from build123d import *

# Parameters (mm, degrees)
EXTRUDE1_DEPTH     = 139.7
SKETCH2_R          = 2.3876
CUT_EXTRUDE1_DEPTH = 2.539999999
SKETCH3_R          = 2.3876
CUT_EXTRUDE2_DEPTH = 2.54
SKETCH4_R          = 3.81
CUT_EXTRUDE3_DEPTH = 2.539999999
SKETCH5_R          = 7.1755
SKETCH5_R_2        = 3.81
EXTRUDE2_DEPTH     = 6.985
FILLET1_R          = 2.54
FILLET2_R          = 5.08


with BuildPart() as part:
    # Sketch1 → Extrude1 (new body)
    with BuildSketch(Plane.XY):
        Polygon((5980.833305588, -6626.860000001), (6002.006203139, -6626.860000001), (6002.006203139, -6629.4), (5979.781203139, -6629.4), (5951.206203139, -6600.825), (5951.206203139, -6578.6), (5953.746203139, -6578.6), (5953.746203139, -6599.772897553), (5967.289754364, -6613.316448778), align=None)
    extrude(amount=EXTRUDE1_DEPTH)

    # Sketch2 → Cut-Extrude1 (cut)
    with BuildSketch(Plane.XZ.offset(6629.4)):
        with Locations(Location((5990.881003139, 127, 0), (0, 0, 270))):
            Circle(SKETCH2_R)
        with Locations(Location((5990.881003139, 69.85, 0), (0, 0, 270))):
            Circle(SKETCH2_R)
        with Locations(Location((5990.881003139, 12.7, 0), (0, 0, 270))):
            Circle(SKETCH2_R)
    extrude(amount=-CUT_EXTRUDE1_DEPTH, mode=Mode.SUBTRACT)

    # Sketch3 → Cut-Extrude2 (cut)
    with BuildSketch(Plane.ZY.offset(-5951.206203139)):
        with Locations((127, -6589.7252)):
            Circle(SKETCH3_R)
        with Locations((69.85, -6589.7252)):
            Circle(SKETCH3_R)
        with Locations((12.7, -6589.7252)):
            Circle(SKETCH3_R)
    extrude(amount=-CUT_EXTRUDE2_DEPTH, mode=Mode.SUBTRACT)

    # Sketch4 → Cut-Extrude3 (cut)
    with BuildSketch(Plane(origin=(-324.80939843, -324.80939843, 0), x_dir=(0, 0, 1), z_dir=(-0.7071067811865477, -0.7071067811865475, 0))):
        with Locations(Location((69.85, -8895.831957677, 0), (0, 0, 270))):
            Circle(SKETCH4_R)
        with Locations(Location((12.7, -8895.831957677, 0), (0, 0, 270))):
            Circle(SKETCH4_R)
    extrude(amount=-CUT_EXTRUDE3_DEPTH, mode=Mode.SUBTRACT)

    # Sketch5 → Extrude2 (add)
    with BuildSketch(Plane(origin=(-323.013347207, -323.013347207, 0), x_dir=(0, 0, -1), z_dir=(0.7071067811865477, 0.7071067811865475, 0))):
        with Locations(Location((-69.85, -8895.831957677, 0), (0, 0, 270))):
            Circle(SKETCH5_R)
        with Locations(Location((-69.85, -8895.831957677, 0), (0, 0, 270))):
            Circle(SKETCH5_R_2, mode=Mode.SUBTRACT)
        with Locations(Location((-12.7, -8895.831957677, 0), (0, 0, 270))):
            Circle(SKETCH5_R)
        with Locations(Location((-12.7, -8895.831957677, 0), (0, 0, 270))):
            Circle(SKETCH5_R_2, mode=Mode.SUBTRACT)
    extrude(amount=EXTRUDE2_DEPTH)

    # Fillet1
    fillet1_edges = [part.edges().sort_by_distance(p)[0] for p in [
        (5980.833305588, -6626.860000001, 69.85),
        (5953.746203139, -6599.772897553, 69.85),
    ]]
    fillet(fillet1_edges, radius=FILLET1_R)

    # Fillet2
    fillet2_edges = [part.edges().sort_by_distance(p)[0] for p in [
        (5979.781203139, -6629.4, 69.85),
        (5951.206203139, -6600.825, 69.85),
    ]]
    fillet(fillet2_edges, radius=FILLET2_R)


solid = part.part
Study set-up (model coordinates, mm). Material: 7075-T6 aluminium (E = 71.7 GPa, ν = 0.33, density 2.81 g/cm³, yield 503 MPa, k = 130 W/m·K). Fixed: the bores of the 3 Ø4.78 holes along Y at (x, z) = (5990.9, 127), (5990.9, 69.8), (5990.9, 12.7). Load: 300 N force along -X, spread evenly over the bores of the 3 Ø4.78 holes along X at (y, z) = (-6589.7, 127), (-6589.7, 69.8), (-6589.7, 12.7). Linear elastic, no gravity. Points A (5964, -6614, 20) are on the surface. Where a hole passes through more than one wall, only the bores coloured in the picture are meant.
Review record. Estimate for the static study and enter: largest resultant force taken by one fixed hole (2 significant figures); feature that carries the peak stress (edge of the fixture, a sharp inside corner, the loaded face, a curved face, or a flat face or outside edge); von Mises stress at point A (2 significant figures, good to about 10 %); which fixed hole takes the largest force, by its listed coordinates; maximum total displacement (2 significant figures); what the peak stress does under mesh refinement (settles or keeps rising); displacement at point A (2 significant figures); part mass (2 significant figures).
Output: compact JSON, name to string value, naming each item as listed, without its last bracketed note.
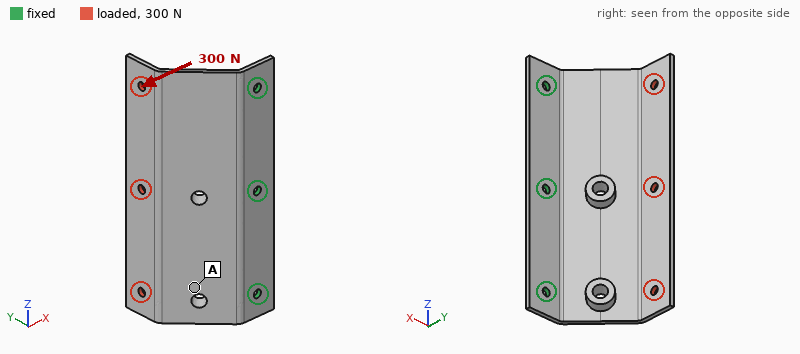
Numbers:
{"largest resultant force taken by one fixed hole": "230 N", "feature that carries the peak stress": "edge of the fixture", "von Mises stress at point A": "21 MPa", "which fixed hole takes the largest force, by its listed coordinates": "(5990.9, 69.8)", "maximum total displacement": "1.5 mm", "what the peak stress does under mesh refinement": "keeps rising", "displacement at point A": "0.45 mm", "part mass": "85 g"}
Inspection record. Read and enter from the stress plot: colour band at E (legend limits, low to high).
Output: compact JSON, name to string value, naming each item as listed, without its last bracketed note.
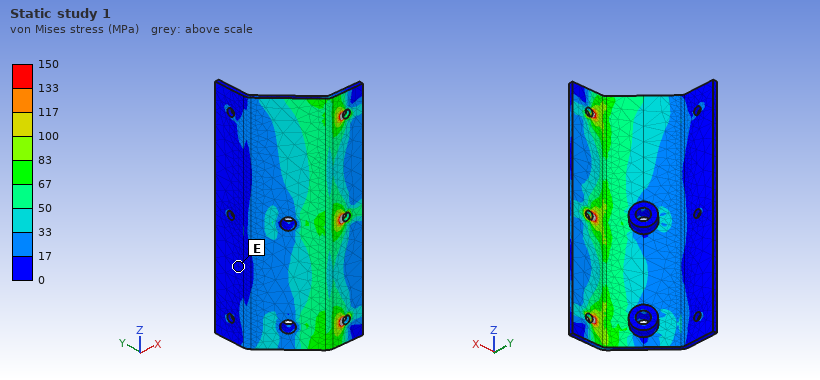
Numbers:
{"colour band at E": "0 to 17 MPa"}
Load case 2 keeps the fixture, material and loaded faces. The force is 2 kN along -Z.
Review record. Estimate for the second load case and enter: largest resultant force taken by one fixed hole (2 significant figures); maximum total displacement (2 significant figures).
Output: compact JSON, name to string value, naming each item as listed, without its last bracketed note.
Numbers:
{"largest resultant force taken by one fixed hole": "1.1 kN", "maximum total displacement": "1.3 mm"}
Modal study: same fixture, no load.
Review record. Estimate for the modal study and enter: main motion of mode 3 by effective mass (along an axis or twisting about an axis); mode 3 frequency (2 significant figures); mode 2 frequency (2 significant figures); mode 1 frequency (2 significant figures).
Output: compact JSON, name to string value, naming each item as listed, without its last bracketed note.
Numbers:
{"main motion of mode 3 by effective mass": "along Y", "mode 3 frequency": "2200 Hz", "mode 2 frequency": "690 Hz", "mode 1 frequency": "420 Hz"}
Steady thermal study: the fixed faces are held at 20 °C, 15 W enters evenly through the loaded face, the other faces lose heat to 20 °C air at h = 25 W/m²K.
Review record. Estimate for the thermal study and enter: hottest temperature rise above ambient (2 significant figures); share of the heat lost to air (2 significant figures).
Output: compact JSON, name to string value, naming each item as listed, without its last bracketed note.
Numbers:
{"hottest temperature rise above ambient": "22 K", "share of the heat lost to air": "37 %"}
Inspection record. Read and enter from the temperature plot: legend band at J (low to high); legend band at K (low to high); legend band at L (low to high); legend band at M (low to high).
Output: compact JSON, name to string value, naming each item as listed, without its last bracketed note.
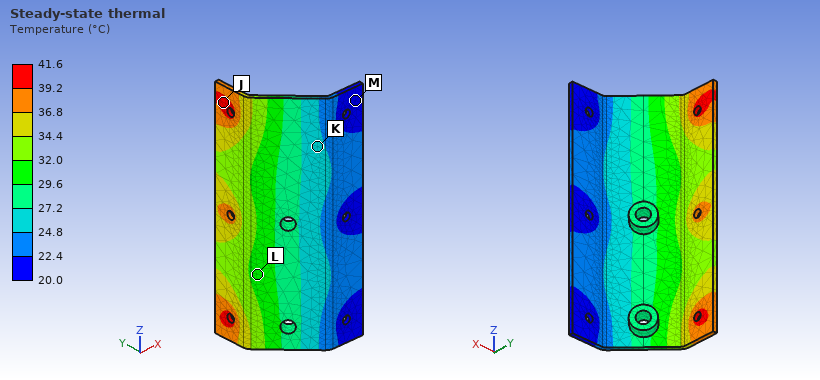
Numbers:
{"legend band at J": "39.2 to 41.6 °C", "legend band at K": "24.8 to 27.2 °C", "legend band at L": "29.6 to 32.0 °C", "legend band at M": "20.0 to 22.4 °C"}
